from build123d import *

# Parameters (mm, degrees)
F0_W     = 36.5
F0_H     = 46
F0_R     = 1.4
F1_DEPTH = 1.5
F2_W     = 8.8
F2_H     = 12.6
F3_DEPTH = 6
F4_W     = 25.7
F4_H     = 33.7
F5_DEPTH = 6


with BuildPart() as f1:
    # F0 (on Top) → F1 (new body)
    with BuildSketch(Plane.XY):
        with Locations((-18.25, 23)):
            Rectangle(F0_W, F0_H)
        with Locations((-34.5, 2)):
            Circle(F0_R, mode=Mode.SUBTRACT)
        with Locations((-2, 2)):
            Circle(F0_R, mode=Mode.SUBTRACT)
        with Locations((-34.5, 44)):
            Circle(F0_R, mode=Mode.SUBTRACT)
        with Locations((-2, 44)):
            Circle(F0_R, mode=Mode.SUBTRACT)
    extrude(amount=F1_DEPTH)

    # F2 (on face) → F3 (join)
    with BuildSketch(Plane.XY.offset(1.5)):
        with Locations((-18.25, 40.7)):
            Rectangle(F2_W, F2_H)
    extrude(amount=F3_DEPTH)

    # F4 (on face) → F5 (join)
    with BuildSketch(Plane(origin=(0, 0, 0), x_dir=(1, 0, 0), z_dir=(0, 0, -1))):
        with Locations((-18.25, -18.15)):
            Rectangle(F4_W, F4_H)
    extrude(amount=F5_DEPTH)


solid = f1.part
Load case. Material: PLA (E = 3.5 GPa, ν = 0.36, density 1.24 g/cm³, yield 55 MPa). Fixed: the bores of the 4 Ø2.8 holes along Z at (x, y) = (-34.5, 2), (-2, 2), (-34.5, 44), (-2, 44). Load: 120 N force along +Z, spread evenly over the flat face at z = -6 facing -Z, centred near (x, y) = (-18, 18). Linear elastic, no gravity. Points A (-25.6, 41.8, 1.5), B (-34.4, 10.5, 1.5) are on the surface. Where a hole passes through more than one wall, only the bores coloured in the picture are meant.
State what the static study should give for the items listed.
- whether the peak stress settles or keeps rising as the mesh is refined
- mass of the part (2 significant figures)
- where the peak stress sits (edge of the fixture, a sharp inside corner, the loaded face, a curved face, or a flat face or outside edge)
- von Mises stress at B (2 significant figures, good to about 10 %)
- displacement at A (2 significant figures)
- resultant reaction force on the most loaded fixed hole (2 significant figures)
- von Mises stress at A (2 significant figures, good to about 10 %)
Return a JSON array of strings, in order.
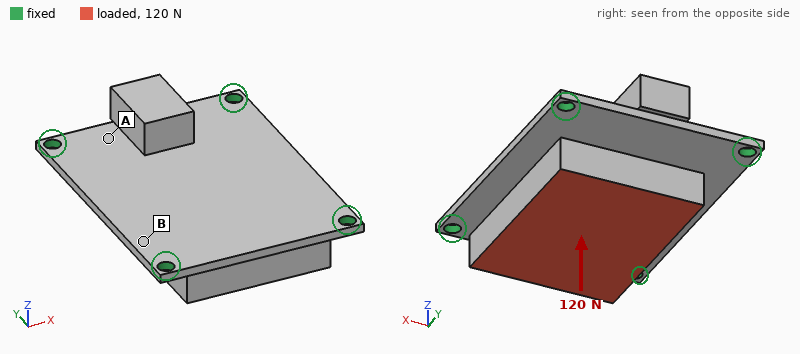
["keeps rising", "10 g", "edge of the fixture", "3.0 MPa", "0.13 mm", "47 N", "7.7 MPa"]
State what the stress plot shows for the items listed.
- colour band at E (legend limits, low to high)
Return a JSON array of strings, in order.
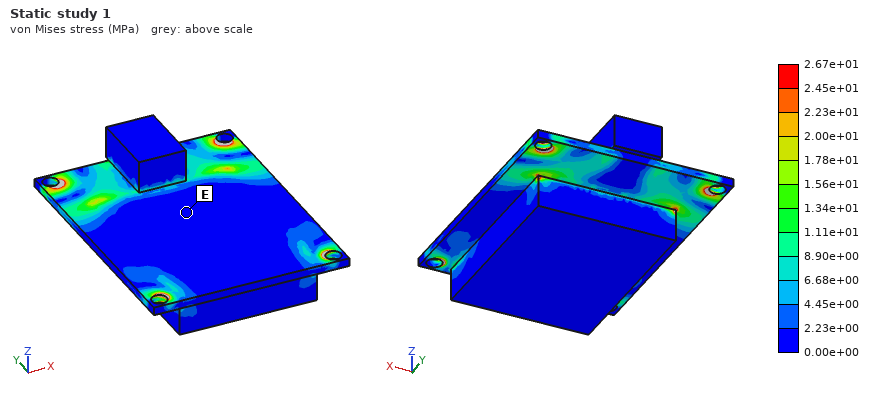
["0.00e+00 to 2.23e+00 MPa"]
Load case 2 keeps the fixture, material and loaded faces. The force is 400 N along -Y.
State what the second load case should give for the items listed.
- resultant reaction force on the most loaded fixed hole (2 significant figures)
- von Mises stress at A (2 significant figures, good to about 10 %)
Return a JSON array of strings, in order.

["130 N", "11 MPa"]
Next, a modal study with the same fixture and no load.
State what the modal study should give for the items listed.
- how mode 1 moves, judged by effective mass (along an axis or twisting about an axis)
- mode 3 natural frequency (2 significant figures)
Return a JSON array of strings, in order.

["along Z", "3200 Hz"]
